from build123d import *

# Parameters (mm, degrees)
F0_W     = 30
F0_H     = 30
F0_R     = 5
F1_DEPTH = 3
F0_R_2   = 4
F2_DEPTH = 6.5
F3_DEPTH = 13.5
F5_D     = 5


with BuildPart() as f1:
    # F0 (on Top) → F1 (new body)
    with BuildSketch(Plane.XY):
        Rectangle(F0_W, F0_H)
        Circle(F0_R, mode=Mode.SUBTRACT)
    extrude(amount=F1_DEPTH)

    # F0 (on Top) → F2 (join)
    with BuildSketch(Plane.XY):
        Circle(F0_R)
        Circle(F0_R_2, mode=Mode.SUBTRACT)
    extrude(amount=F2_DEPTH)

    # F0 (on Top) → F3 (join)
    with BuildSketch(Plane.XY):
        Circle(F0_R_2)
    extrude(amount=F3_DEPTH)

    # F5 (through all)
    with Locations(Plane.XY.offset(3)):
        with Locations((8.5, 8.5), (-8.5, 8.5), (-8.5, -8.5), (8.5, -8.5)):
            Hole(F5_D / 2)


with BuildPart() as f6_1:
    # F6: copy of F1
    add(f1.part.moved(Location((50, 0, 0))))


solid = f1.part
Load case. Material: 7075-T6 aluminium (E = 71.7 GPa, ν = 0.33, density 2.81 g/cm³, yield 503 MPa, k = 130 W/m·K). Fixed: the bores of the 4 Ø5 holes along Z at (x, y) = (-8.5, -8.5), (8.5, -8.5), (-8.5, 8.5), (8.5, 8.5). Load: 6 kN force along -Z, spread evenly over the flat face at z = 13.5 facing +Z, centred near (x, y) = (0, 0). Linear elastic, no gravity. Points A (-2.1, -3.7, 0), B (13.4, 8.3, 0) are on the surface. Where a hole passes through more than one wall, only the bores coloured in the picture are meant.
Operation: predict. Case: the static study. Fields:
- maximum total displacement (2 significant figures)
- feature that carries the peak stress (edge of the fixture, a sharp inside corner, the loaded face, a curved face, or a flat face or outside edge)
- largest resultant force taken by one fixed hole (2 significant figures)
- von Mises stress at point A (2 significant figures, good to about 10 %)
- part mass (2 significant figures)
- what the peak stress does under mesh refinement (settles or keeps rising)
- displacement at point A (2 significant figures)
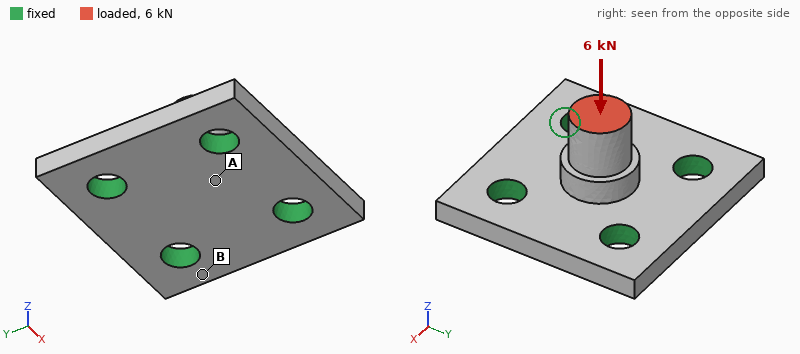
53 µm
edge of the fixture
1.6 kN
150 MPa
8.7 g
keeps rising
35 µm
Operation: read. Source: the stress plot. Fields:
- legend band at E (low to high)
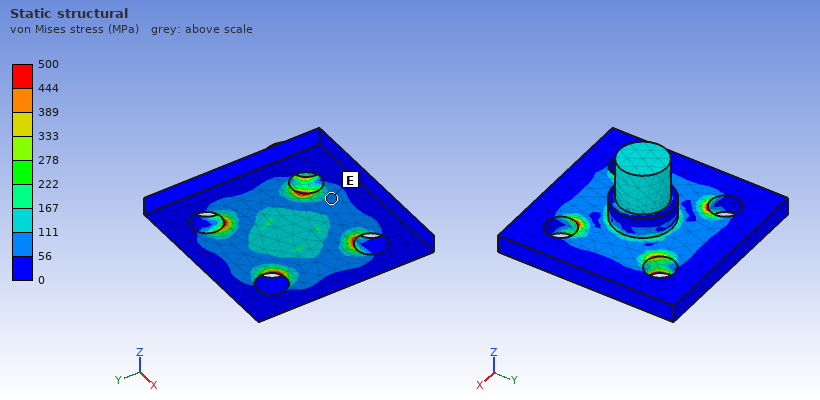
56 to 111 MPa
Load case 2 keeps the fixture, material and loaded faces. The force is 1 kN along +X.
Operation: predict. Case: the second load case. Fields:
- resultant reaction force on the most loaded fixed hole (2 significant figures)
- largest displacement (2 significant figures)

540 N
56 µm
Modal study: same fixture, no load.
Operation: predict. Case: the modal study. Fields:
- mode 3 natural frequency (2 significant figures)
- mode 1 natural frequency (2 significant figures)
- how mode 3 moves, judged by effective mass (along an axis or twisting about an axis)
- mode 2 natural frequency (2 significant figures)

36 kHz
29 kHz
along Z
30 kHz
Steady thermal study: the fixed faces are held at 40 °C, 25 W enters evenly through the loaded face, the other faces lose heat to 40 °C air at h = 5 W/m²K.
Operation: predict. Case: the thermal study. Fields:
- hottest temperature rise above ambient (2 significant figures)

49 K
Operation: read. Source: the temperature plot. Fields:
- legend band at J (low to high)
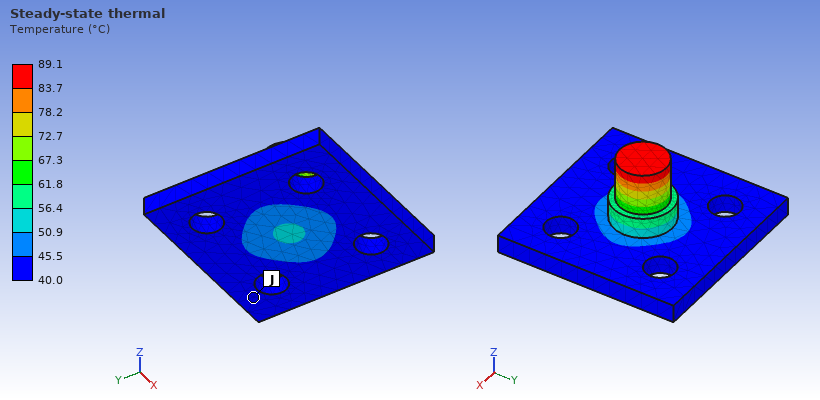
40.0 to 45.5 °C
